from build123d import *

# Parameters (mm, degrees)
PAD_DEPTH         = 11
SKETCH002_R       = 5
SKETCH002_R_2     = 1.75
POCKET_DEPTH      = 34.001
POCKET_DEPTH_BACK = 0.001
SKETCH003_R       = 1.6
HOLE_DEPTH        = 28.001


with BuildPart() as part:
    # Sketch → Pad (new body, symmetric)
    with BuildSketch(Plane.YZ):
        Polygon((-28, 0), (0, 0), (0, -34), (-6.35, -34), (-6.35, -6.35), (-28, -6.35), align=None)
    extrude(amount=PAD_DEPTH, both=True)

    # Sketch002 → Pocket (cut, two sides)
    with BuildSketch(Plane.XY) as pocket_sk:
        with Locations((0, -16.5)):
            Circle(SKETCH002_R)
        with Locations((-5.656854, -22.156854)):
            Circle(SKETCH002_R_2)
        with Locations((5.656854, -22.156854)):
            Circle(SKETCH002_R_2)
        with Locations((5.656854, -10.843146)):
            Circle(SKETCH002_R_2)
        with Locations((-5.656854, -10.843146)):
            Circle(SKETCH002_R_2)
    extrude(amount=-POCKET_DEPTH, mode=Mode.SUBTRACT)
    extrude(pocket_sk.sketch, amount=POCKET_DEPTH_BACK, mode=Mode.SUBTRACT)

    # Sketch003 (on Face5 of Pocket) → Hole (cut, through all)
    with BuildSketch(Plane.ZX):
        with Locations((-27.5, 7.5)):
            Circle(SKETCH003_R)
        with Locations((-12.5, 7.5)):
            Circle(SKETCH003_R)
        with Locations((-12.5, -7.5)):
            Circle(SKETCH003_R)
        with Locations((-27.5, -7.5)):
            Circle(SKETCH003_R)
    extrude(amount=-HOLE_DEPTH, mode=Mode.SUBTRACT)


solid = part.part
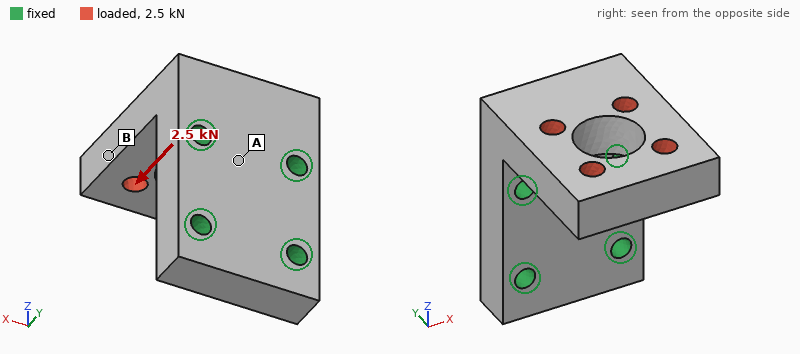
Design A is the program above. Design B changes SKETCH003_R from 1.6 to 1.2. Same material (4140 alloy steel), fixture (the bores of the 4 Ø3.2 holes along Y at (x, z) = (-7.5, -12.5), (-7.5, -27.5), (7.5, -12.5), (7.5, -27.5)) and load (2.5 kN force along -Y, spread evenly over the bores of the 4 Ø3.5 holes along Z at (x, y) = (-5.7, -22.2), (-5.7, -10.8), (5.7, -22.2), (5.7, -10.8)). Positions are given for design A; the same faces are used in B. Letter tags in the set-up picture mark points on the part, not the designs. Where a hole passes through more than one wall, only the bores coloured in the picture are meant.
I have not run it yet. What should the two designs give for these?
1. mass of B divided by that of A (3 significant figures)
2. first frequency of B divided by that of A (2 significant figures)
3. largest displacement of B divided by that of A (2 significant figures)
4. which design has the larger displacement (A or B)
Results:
1.01
0.98
1.1
B
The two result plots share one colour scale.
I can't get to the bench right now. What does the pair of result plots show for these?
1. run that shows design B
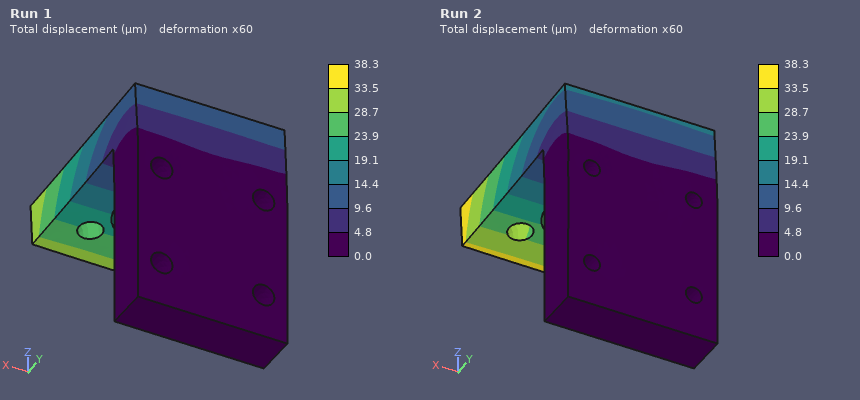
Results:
Run 2
